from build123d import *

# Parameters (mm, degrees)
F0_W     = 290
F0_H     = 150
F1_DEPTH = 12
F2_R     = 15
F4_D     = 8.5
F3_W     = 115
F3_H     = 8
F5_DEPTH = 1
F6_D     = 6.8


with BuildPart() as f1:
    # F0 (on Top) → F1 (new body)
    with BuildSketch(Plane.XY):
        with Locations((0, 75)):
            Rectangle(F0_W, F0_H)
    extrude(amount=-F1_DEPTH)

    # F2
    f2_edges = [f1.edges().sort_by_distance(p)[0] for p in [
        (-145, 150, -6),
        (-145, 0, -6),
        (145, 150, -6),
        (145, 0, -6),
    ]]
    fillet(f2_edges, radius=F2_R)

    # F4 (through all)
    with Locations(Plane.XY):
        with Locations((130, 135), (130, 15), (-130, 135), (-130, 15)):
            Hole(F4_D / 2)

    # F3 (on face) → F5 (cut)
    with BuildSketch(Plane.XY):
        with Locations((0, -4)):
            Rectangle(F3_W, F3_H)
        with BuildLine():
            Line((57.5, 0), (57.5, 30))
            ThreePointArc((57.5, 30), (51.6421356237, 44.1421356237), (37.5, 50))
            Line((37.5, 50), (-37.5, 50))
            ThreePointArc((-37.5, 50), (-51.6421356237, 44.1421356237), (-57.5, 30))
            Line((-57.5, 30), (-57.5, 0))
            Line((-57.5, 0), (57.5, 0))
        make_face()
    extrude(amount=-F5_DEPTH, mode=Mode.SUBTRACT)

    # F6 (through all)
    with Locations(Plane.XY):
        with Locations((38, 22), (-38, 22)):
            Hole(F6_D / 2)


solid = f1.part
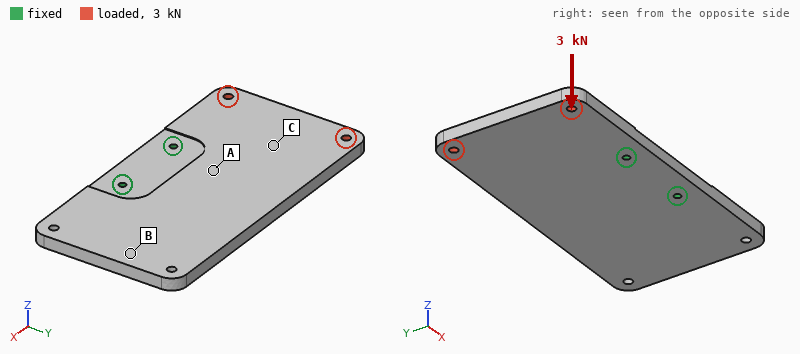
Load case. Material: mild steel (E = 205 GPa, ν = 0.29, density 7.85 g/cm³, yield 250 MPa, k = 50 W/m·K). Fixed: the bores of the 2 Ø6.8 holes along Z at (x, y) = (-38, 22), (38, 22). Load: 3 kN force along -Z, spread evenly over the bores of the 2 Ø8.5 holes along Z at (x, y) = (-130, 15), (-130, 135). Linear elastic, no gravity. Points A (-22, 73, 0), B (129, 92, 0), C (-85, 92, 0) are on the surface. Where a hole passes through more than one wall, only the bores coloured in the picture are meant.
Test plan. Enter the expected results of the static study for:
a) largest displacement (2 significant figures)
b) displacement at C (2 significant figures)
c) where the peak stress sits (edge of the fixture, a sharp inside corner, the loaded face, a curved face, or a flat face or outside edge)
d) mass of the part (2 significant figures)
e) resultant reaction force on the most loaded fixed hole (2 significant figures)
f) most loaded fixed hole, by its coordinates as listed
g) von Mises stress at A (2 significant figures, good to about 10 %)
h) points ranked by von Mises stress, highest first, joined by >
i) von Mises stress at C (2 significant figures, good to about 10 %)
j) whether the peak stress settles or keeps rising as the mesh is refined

0.70 mm
0.29 mm
edge of the fixture
4.0 kg
5.0 kN
(-38, 22)
58 MPa
A > C > B
31 MPa
keeps rising
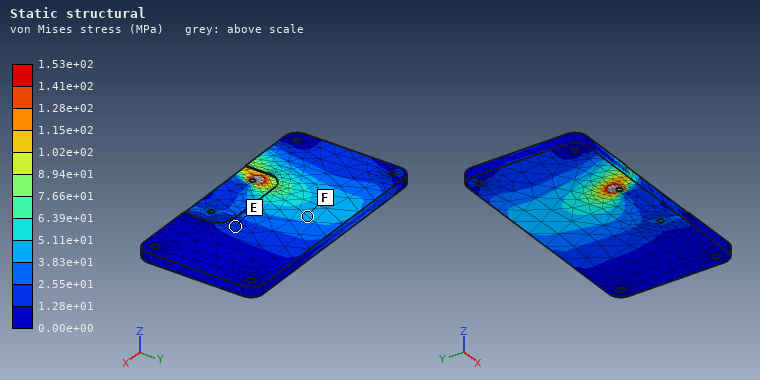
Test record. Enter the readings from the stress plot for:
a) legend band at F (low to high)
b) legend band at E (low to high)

3.83e+01 to 5.11e+01 MPa
1.28e+01 to 2.55e+01 MPa
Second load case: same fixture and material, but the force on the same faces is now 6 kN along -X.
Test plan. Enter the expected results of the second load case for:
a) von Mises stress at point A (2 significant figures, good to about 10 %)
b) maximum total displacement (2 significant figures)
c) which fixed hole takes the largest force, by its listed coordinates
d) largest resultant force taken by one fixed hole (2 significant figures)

5.6 MPa
16 µm
(-38, 22)
5.5 kN
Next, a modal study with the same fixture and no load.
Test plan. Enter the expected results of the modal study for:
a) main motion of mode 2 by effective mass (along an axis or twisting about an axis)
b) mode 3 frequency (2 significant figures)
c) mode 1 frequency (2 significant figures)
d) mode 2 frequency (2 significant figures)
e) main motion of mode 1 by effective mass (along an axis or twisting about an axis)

twisting about Y
760 Hz
380 Hz
450 Hz
along Z
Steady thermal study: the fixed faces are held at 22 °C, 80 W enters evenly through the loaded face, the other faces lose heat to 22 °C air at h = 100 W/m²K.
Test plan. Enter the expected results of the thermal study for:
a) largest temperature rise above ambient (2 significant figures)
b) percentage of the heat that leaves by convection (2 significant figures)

58 K
91 %
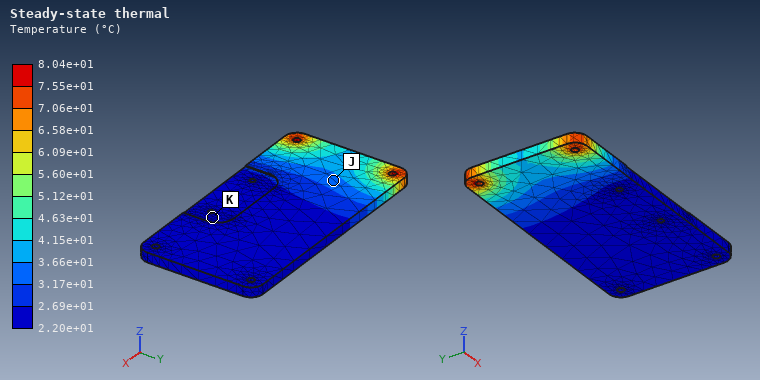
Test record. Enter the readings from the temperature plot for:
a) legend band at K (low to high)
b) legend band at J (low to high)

2.20e+01 to 2.69e+01 °C
3.17e+01 to 3.66e+01 °C
